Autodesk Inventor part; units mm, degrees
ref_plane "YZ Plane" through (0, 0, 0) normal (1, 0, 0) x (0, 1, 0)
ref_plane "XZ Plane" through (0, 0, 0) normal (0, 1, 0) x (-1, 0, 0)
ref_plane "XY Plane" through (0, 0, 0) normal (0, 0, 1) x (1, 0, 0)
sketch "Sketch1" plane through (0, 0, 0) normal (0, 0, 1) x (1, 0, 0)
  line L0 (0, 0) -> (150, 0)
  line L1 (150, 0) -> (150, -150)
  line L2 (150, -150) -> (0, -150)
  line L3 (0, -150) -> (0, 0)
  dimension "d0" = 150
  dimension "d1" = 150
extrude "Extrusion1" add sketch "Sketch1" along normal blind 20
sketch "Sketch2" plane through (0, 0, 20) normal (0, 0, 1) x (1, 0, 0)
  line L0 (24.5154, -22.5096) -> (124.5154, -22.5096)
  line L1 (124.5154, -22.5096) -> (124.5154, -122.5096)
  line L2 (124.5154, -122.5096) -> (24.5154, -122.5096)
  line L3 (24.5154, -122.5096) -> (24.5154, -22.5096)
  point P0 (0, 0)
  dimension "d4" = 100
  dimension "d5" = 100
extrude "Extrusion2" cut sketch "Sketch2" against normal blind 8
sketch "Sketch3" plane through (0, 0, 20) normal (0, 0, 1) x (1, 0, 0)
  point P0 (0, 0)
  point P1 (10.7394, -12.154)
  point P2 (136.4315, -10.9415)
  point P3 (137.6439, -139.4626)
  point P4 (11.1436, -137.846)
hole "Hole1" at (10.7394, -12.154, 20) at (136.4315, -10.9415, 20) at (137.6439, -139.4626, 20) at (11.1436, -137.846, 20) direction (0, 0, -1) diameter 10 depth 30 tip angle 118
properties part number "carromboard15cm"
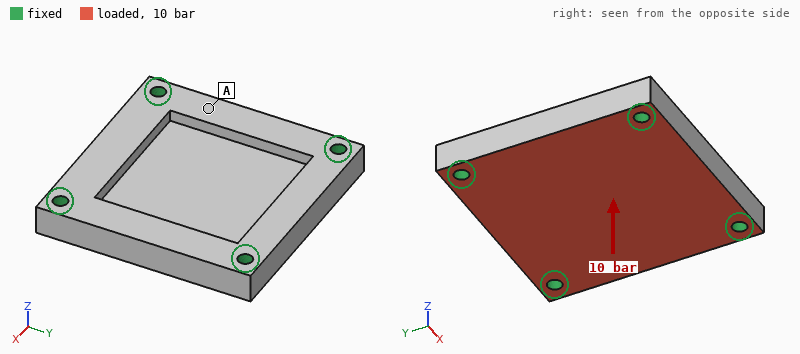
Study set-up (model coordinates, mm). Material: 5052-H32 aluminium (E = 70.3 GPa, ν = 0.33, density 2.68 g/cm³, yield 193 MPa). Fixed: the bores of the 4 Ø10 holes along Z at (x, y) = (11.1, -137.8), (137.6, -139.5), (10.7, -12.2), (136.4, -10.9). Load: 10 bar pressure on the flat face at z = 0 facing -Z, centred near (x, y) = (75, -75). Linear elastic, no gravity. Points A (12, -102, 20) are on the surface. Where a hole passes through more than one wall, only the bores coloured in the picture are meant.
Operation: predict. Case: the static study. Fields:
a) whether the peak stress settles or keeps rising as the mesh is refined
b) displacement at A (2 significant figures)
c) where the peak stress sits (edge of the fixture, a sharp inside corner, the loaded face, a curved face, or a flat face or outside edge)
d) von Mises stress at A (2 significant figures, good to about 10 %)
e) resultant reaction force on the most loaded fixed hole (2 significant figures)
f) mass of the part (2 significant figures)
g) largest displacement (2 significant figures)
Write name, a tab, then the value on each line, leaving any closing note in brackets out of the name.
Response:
whether the peak stress settles or keeps rising as the mesh is refined	keeps rising
displacement at A	25 µm
where the peak stress sits	edge of the fixture
von Mises stress at A	10 MPa
resultant reaction force on the most loaded fixed hole	6.0 kN
mass of the part	970 g
largest displacement	81 µm
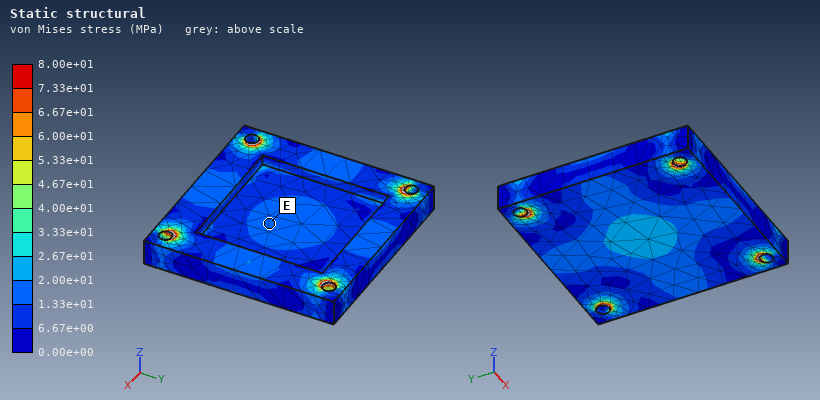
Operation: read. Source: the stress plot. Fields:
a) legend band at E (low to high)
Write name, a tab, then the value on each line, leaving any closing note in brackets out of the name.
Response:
legend band at E	1.33e+01 to 2.00e+01 MPa
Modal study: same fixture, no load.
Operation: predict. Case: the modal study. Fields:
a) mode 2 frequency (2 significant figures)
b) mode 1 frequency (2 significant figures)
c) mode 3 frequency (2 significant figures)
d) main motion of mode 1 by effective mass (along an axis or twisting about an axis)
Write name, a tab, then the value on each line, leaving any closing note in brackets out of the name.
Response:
mode 2 frequency	5800 Hz
mode 1 frequency	3700 Hz
mode 3 frequency	5900 Hz
main motion of mode 1 by effective mass	along Z
